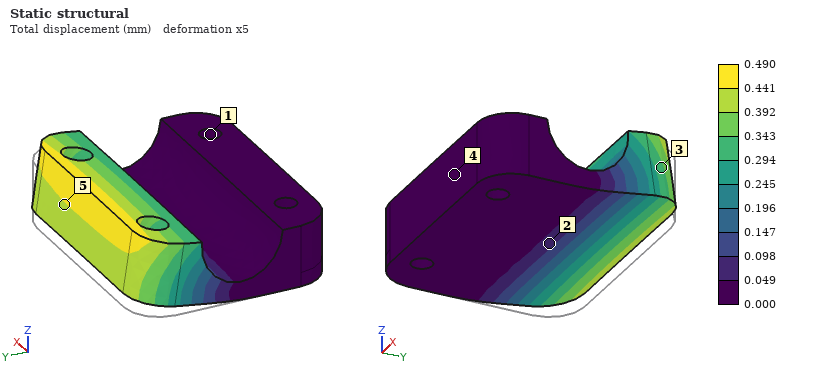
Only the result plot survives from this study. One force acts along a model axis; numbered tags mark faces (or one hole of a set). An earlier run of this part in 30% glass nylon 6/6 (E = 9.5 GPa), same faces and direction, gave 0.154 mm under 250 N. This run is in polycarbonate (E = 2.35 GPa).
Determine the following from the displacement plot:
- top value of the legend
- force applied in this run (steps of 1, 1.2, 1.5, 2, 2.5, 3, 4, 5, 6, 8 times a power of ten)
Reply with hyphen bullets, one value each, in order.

- 0.490 mm
- 200 N
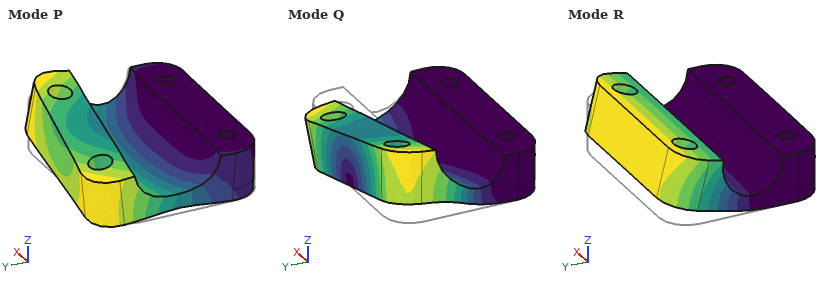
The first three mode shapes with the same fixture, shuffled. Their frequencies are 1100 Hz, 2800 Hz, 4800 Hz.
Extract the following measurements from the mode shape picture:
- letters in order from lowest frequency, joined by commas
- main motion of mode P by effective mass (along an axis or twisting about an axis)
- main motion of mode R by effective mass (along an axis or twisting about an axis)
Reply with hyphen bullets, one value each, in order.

- R, Q, P
- along X
- along Z
